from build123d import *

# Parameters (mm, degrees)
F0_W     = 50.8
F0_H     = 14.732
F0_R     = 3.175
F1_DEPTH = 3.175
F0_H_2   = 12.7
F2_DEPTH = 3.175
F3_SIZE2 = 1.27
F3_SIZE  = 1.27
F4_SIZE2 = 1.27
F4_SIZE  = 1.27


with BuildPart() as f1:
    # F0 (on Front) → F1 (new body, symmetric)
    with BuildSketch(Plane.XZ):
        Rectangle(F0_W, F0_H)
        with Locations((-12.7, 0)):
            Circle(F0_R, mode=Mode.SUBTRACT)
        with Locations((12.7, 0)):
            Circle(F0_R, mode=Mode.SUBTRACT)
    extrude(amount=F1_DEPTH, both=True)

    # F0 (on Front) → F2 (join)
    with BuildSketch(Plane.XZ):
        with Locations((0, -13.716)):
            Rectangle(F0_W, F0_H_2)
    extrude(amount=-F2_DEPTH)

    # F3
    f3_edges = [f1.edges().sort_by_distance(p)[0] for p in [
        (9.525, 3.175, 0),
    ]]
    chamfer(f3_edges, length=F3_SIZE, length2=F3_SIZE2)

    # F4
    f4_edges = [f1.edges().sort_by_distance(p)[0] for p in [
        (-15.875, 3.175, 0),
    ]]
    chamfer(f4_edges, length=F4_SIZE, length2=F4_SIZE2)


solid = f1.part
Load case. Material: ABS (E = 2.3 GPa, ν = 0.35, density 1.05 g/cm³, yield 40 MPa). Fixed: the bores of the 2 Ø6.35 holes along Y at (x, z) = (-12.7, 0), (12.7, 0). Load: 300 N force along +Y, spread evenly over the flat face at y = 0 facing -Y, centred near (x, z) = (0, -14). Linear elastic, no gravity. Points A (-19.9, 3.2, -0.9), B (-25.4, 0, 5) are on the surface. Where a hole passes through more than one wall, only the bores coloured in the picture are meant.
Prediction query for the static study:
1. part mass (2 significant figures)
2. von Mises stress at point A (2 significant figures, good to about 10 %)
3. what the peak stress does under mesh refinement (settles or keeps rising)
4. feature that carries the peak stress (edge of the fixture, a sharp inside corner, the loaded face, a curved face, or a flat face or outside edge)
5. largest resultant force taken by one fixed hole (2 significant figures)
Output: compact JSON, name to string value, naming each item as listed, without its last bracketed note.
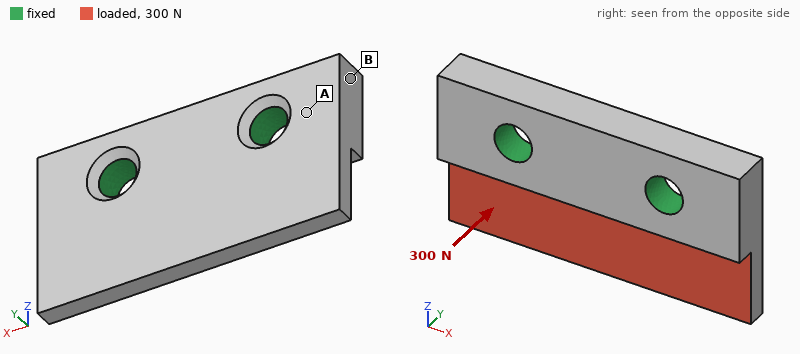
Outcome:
{"part mass": "6.7 g", "von Mises stress at point A": "5.7 MPa", "what the peak stress does under mesh refinement": "keeps rising", "feature that carries the peak stress": "edge of the fixture", "largest resultant force taken by one fixed hole": "150 N"}
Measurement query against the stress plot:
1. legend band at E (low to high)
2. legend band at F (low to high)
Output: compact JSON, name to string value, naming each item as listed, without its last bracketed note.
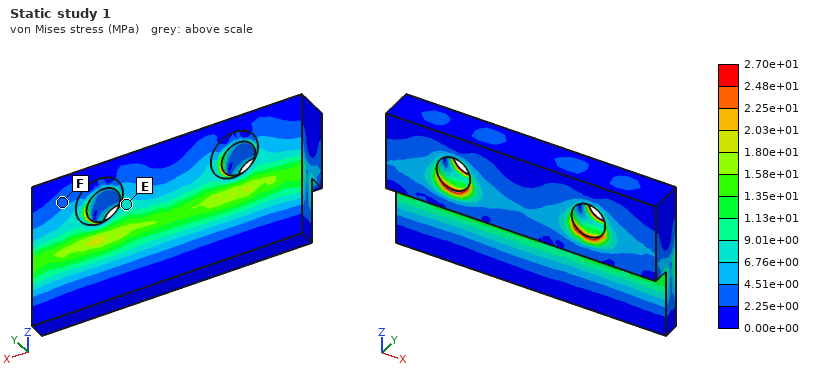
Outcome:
{"legend band at E": "6.76e+00 to 9.01e+00 MPa", "legend band at F": "2.25e+00 to 4.51e+00 MPa"}
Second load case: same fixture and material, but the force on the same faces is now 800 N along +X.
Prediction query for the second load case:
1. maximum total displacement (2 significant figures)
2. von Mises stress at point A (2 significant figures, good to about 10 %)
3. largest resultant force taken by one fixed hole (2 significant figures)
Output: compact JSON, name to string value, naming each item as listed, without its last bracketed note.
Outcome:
{"maximum total displacement": "0.27 mm", "von Mises stress at point A": "5.7 MPa", "largest resultant force taken by one fixed hole": "500 N"}
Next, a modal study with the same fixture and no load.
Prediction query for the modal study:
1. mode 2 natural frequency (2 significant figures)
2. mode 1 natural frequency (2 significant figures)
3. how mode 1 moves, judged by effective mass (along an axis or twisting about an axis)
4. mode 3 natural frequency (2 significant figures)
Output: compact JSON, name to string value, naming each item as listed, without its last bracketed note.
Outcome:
{"mode 2 natural frequency": "3700 Hz", "mode 1 natural frequency": "3200 Hz", "how mode 1 moves, judged by effective mass": "along Y", "mode 3 natural frequency": "4900 Hz"}
